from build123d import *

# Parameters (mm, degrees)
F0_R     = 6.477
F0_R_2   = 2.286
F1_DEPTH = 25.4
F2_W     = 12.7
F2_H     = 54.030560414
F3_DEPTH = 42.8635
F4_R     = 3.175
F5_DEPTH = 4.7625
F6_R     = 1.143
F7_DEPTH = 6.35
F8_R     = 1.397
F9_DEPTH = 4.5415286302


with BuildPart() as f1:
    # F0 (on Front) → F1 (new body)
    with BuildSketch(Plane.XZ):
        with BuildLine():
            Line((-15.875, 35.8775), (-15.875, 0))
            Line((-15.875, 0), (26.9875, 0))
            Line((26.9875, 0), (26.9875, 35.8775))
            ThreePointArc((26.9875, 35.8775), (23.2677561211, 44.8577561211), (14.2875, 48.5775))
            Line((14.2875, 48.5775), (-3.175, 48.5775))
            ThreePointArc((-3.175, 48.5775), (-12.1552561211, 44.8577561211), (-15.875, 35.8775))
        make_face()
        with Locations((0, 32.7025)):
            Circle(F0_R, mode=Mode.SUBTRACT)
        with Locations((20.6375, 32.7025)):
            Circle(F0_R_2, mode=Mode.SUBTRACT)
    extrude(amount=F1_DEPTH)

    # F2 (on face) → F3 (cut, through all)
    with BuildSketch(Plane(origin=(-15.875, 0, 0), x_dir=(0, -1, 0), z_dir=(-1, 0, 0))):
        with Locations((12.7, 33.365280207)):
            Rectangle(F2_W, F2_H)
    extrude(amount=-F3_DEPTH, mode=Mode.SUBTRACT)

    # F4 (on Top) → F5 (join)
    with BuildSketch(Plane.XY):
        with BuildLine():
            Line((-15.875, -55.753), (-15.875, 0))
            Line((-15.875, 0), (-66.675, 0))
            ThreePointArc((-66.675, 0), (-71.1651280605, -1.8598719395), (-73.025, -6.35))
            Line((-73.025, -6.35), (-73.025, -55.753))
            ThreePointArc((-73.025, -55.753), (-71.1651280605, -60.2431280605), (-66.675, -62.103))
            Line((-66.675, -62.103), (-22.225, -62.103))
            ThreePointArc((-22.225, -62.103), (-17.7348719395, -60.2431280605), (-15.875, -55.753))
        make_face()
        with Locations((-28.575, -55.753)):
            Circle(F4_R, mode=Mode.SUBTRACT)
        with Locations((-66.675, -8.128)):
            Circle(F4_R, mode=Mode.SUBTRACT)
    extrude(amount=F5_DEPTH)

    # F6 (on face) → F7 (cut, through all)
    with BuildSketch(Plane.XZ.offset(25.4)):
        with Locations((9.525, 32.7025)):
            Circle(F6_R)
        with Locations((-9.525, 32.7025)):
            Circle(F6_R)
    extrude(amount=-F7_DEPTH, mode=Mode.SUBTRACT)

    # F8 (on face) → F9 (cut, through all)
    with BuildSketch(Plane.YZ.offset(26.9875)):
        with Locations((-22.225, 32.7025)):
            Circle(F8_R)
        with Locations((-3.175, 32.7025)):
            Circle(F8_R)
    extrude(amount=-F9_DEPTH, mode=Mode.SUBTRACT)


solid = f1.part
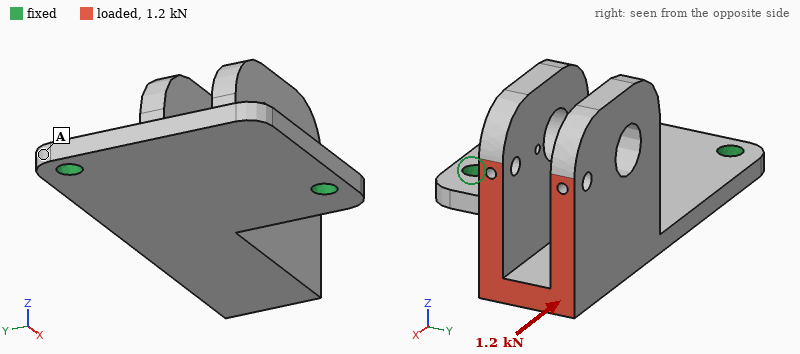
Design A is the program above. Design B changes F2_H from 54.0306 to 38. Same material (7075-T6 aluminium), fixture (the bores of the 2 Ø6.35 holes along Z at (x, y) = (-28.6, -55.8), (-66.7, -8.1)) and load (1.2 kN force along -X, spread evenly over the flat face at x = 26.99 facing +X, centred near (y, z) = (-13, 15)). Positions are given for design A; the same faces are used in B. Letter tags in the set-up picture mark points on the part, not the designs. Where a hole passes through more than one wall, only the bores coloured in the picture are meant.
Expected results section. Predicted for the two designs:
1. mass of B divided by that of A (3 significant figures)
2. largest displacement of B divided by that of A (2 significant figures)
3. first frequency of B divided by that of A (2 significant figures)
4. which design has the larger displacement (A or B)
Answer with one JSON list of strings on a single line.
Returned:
["1.10", "0.91", "0.95", "A"]
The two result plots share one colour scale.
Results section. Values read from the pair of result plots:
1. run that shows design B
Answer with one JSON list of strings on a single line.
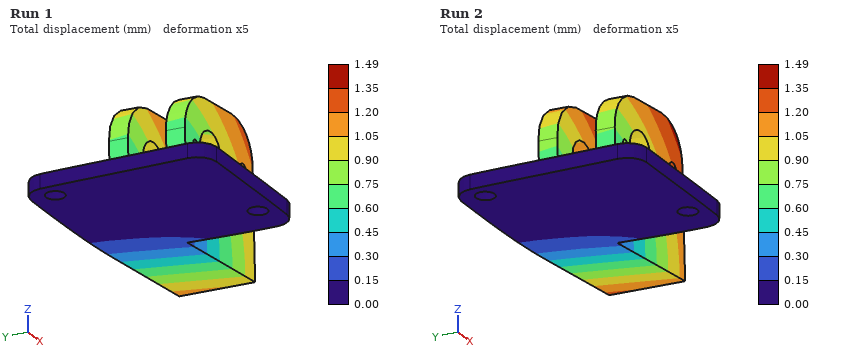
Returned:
["Run 1"]
